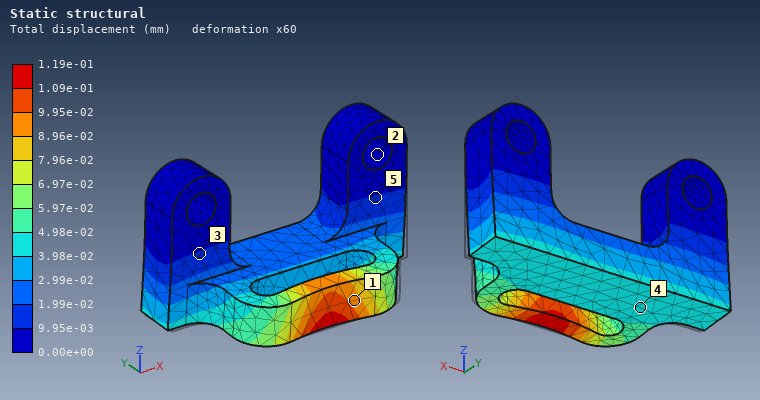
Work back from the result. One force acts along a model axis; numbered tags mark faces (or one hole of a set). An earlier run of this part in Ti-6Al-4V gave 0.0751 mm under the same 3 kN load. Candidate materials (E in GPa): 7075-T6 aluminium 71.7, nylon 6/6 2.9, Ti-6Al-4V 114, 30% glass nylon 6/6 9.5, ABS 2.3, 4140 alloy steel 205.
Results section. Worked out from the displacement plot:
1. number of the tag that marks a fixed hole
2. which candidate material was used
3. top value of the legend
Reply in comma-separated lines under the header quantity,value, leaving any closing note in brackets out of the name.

quantity,value
number of the tag that marks a fixed hole,2
which candidate material was used,7075-T6 aluminium
top value of the legend,1.19e-01 mm
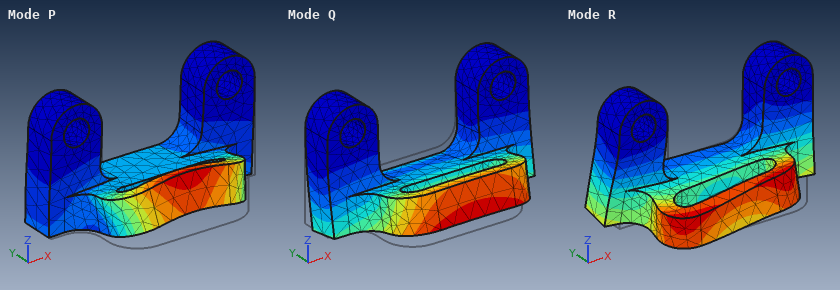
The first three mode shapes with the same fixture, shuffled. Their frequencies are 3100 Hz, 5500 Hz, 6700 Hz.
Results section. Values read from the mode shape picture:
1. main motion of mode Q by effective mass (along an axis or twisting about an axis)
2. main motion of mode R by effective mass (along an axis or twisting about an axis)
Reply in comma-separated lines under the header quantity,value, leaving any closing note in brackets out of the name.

quantity,value
main motion of mode Q by effective mass,along Y
main motion of mode R by effective mass,along X
